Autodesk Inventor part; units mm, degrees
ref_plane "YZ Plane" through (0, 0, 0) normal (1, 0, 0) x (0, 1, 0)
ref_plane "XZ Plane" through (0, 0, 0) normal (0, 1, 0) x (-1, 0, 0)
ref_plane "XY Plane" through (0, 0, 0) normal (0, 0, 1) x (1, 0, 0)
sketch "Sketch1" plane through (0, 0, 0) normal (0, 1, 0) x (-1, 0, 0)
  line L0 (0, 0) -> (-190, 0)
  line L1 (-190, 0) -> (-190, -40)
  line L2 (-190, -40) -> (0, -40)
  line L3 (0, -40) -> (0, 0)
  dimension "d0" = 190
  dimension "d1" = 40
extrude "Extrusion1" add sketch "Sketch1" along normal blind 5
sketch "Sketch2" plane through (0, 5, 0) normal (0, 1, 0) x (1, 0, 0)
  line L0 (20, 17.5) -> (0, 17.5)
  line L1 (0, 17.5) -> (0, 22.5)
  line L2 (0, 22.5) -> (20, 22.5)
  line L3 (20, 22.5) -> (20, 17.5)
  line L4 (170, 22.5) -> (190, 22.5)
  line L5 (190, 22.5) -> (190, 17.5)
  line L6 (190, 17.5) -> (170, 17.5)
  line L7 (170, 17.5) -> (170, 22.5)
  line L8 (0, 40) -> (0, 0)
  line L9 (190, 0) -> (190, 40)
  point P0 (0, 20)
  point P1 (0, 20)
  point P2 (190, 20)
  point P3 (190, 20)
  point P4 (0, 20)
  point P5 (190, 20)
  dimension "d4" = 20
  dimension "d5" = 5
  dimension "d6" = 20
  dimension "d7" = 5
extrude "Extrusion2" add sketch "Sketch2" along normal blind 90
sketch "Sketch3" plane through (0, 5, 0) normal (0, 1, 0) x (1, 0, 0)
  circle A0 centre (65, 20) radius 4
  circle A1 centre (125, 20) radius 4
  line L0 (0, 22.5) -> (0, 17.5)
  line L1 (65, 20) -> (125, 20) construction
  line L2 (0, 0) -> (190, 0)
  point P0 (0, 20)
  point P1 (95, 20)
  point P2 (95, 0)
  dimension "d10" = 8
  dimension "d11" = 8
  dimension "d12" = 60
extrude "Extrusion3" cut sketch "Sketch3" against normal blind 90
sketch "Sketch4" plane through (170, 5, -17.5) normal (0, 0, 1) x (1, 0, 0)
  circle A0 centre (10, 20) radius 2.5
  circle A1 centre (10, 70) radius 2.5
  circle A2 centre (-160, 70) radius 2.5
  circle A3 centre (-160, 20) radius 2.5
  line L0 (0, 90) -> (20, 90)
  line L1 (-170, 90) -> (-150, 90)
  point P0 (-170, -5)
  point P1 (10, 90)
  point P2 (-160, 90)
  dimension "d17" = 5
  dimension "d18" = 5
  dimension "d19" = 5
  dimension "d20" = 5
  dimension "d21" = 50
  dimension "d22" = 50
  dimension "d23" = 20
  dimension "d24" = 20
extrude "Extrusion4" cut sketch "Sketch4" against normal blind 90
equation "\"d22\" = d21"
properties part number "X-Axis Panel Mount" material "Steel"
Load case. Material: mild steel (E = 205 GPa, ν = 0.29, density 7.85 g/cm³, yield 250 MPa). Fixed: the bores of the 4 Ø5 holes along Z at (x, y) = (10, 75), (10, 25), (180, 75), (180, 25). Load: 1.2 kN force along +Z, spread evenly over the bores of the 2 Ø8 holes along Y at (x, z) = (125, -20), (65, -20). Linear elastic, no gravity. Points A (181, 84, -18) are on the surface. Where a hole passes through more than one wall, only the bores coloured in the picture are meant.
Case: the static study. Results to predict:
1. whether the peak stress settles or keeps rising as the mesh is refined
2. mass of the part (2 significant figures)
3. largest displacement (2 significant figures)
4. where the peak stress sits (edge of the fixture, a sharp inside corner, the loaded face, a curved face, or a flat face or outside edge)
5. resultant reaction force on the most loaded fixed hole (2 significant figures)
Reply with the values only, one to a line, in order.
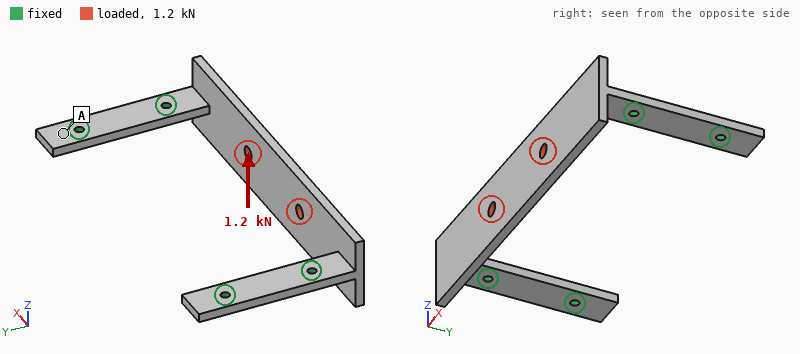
keeps rising
430 g
0.10 mm
edge of the fixture
620 N
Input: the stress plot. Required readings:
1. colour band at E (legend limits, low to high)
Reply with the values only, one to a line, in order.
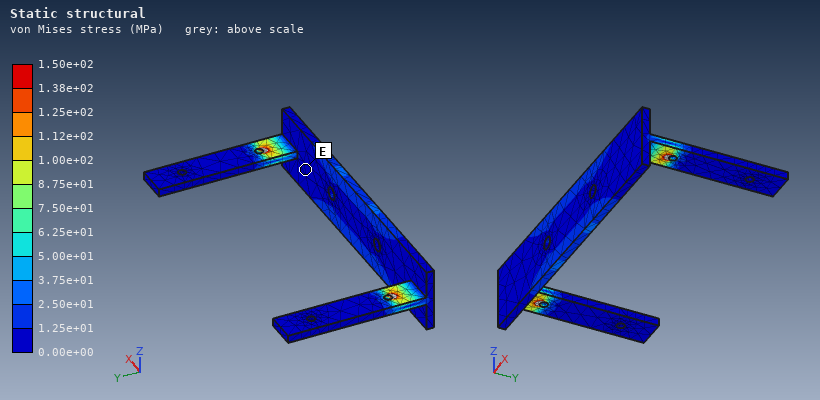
0.00e+00 to 1.25e+01 MPa
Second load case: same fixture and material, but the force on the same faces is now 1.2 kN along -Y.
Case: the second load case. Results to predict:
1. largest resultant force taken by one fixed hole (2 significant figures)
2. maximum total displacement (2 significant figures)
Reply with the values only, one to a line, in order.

1.1 kN
0.23 mm
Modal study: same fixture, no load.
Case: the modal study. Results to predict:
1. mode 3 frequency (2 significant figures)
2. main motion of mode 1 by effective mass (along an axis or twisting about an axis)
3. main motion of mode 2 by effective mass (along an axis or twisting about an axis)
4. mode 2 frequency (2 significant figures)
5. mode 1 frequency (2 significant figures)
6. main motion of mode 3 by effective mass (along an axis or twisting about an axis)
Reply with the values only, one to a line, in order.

2100 Hz
along Y
along Z
1000 Hz
970 Hz
twisting about Y
